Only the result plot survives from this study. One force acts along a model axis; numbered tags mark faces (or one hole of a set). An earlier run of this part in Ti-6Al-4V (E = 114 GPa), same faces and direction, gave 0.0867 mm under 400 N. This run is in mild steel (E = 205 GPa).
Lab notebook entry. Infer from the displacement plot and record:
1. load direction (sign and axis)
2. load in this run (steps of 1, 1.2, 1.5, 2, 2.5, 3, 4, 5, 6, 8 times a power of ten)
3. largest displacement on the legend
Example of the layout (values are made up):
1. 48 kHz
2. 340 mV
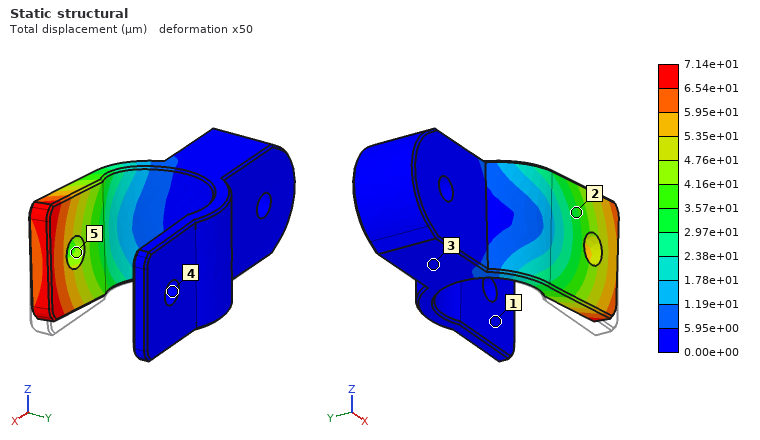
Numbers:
1. +Z
2. 600 N
3. 7.14e+01 µm
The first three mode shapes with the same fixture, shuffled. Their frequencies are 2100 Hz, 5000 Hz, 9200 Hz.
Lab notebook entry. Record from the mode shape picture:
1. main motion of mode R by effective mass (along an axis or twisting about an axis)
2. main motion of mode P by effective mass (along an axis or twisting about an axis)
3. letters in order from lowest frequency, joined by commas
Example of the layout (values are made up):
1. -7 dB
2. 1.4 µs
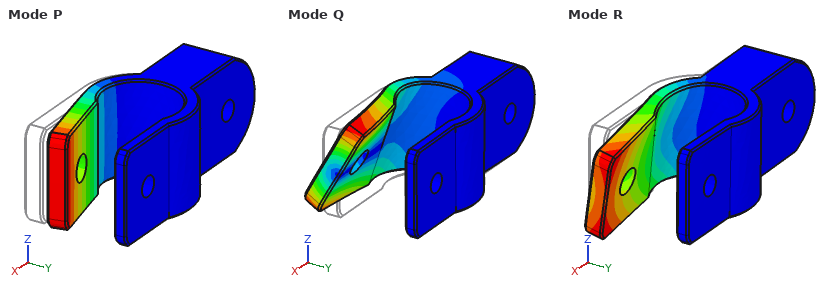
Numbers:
1. along Z
2. along Y
3. P, R, Q
